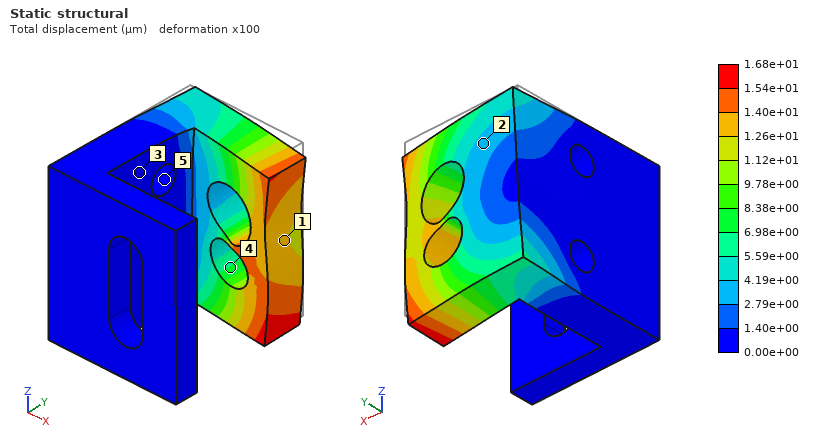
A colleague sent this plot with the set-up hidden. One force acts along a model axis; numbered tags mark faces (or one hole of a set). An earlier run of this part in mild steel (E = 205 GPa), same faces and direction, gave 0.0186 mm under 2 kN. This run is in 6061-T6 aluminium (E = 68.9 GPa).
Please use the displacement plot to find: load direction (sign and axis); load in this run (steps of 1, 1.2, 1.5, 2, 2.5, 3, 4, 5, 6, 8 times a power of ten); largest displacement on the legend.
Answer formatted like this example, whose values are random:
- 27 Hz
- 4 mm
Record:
- -Z
- 600 N
- 1.68e+01 µm
